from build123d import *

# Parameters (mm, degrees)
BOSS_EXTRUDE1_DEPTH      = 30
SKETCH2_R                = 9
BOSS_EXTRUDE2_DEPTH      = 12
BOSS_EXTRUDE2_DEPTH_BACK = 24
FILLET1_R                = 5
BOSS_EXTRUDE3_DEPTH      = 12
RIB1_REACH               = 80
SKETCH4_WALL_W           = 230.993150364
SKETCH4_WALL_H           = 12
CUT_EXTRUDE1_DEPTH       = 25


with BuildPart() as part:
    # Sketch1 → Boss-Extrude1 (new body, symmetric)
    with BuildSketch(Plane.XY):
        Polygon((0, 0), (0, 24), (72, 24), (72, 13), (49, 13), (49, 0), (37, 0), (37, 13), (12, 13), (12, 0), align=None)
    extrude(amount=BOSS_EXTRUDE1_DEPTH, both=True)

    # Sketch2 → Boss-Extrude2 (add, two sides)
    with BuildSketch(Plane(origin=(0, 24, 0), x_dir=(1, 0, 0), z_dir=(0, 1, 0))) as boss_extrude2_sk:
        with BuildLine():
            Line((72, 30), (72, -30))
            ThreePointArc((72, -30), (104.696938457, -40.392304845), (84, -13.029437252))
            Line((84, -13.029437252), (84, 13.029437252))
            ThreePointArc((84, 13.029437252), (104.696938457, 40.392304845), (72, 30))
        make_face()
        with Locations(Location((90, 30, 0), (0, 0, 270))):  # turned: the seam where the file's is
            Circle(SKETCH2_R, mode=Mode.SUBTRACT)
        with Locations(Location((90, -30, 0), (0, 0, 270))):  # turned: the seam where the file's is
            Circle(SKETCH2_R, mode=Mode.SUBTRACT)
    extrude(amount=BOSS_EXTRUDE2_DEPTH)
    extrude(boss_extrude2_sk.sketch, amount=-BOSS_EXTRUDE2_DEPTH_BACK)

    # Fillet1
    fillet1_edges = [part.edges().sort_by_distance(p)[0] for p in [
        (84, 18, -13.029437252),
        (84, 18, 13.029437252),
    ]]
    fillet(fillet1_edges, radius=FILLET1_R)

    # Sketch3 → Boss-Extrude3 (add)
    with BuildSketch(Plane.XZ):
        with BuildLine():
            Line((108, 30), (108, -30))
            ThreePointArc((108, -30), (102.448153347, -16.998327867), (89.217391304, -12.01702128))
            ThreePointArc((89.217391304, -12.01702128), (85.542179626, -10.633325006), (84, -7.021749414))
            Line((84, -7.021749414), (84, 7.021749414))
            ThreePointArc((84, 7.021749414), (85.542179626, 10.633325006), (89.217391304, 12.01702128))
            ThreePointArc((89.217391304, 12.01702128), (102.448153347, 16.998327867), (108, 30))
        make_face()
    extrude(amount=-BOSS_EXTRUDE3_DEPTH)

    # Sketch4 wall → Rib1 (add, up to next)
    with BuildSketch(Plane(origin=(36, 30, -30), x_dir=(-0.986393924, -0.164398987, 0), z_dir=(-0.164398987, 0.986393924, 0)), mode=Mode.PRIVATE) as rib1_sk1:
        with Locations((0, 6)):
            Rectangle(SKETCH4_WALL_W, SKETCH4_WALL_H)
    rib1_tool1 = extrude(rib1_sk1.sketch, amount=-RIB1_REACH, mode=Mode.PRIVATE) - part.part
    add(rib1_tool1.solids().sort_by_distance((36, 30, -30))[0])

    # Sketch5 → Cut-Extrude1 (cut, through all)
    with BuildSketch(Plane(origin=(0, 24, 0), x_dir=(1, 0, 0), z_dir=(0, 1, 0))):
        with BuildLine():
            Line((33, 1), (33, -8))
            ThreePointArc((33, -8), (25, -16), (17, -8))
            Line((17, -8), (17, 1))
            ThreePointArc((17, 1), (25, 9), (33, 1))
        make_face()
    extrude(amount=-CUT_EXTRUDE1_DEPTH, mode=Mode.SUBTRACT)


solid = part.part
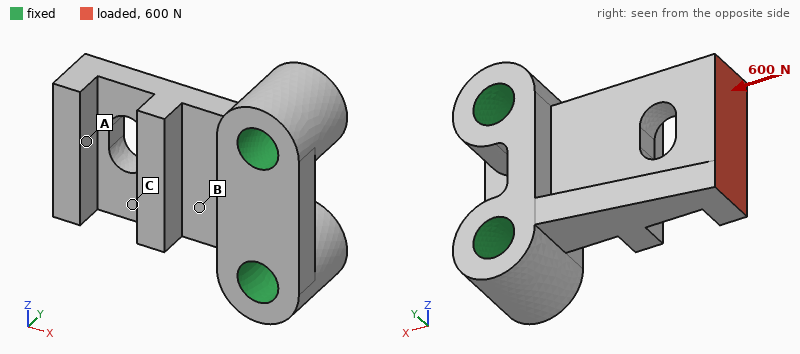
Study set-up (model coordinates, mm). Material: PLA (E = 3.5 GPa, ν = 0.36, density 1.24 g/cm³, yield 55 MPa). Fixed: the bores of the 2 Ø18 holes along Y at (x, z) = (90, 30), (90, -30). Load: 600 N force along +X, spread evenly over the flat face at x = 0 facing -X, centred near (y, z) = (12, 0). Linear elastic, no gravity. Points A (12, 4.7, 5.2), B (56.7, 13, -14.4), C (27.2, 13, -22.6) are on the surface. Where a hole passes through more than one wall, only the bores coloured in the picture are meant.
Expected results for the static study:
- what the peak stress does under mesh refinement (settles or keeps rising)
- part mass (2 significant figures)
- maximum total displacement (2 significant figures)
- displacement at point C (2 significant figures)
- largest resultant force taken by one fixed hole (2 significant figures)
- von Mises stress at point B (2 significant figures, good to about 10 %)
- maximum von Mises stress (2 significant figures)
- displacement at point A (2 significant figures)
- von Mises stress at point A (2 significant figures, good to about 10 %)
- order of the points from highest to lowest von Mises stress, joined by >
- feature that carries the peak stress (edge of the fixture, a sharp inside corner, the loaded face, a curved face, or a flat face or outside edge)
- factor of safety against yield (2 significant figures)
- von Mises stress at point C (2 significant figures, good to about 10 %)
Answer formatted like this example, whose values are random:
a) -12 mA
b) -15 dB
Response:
a) settles
b) 180 g
c) 0.39 mm
d) 0.11 mm
e) 320 N
f) 2.9 MPa
g) 11 MPa
h) 0.26 mm
i) 1.1 MPa
j) C > B > A
k) a curved face
l) 5.2
m) 4.9 MPa
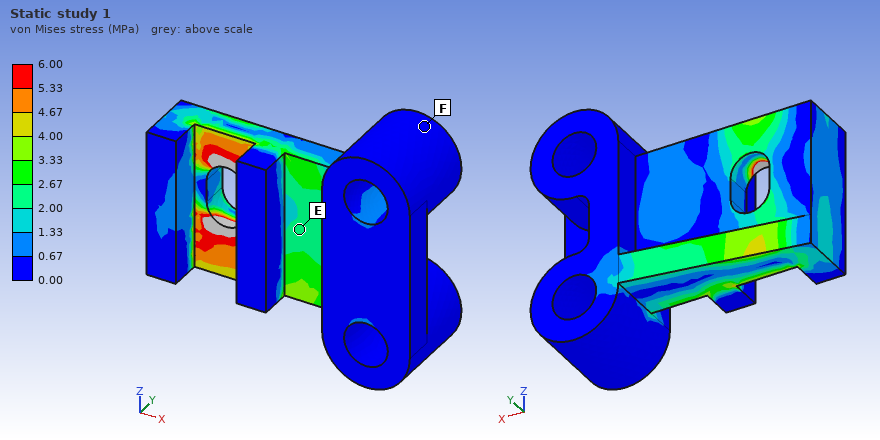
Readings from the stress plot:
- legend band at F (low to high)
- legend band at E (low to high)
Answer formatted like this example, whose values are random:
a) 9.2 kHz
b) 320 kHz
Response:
a) 0.00 to 0.67 MPa
b) 2.00 to 2.67 MPa
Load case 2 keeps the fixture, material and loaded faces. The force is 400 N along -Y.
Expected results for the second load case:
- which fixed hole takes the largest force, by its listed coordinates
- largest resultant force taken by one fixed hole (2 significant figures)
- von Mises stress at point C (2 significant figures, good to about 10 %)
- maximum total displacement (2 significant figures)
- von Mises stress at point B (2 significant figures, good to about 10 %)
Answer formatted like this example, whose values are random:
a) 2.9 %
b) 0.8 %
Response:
a) (90, -30)
b) 230 N
c) 11 MPa
d) 1.6 mm
e) 11 MPa
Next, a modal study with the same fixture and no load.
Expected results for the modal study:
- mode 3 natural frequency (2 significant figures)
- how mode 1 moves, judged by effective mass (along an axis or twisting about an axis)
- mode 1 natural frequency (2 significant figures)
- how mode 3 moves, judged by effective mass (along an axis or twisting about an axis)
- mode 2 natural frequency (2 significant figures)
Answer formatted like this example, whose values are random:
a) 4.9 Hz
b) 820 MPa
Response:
a) 1600 Hz
b) along Y
c) 560 Hz
d) along Z
e) 1300 Hz
